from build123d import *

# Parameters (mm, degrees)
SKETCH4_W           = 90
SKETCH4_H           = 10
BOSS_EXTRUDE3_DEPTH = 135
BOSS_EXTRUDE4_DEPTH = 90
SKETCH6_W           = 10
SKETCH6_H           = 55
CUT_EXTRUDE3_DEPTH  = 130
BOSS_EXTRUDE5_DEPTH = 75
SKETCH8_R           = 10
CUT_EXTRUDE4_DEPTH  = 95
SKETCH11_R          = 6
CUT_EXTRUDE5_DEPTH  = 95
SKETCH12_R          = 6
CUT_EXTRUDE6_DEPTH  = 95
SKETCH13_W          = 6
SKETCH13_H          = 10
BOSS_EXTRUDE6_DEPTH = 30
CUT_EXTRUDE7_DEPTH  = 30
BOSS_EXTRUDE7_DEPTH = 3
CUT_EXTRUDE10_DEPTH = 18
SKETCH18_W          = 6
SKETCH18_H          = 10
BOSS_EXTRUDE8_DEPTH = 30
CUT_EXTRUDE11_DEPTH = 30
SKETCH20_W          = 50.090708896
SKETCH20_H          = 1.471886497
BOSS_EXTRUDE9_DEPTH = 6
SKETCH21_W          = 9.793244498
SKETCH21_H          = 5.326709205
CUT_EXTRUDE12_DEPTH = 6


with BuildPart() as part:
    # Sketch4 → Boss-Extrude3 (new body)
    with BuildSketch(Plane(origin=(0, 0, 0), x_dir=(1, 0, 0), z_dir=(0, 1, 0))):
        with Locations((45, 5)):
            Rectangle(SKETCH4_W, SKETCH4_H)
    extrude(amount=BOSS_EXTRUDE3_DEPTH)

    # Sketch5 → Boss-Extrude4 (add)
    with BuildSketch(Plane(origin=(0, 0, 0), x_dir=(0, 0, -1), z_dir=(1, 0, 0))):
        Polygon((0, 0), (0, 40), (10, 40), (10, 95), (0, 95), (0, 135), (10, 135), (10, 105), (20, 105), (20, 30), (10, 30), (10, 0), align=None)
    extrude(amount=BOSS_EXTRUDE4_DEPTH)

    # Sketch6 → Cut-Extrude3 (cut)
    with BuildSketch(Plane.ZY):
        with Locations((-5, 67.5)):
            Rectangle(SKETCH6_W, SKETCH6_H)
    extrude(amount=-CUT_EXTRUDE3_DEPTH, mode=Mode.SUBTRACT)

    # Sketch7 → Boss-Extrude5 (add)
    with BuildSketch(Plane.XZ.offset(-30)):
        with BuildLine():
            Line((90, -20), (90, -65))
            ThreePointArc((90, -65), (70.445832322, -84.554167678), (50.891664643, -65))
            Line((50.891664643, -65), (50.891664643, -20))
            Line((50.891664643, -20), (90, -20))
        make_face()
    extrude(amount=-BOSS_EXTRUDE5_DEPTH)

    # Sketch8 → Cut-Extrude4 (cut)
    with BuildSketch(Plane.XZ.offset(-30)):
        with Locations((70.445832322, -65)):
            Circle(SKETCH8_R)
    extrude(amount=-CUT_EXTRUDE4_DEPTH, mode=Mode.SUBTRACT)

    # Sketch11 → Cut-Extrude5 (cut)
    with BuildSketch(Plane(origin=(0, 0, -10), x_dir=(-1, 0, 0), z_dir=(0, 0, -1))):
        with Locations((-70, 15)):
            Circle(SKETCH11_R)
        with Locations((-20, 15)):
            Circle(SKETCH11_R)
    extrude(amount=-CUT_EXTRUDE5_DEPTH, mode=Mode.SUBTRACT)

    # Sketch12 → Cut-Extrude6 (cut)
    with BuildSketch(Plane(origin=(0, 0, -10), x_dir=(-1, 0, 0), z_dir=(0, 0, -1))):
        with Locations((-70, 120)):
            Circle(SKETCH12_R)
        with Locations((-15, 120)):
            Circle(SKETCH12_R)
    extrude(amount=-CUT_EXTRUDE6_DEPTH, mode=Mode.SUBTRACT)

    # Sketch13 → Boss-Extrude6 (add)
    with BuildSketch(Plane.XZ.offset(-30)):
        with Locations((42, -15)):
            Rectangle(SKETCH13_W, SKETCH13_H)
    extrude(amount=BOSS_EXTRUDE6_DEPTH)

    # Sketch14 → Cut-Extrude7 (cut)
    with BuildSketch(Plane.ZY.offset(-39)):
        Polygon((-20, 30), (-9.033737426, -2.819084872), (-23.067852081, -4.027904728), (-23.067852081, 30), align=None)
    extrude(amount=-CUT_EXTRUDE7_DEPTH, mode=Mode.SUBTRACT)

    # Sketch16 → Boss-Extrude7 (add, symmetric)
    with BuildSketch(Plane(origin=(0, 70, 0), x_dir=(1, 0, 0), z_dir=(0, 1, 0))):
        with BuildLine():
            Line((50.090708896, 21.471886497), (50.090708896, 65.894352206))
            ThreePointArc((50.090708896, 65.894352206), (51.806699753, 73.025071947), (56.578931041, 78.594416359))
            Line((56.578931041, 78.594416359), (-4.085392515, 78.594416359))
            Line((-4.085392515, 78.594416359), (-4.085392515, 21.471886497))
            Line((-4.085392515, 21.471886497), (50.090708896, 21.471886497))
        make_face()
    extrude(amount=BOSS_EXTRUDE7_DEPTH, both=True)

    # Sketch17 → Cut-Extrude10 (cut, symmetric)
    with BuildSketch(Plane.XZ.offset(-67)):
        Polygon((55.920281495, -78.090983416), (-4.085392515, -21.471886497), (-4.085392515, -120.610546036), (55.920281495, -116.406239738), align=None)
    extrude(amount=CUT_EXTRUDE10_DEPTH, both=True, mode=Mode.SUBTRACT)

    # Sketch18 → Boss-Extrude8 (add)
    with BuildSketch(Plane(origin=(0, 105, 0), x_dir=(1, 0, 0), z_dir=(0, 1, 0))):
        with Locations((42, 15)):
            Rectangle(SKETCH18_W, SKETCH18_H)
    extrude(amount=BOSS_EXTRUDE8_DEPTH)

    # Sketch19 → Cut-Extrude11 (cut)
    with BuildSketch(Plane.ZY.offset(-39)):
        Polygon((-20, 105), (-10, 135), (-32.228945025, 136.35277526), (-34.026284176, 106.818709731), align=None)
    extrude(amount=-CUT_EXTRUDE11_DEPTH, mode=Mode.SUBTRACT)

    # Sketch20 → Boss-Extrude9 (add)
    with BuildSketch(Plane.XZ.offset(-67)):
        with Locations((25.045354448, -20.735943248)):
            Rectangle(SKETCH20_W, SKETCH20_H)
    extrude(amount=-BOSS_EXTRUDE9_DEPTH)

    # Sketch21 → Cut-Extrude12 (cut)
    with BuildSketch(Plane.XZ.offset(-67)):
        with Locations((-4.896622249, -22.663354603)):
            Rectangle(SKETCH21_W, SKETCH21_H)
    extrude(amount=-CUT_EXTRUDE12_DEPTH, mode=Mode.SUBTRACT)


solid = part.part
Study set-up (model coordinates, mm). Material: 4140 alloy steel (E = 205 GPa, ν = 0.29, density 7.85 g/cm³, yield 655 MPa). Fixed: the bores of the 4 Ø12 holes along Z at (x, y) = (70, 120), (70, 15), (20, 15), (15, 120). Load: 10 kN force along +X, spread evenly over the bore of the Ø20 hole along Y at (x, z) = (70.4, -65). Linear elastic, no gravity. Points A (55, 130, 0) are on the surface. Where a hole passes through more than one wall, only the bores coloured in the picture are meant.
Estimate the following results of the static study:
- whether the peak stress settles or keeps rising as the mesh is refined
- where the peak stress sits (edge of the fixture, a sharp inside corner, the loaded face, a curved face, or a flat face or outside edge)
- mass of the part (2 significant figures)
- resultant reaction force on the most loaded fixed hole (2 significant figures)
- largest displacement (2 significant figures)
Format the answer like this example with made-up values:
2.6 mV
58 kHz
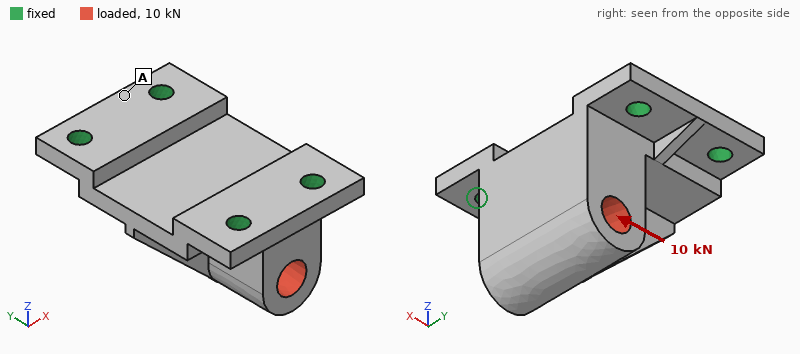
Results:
keeps rising
edge of the fixture
2.3 kg
9.2 kN
84 µm
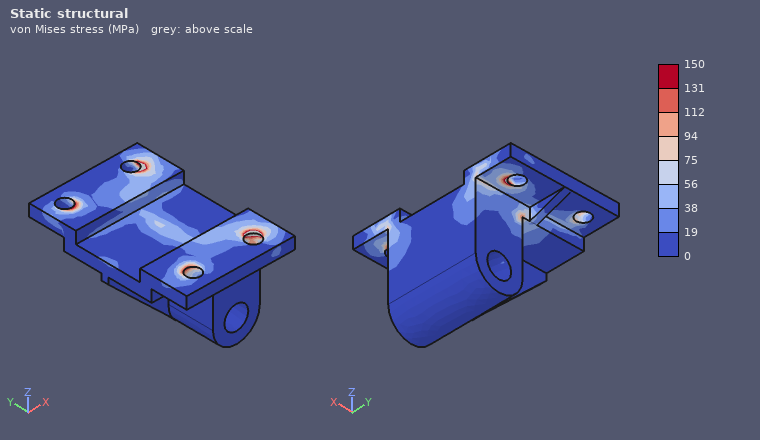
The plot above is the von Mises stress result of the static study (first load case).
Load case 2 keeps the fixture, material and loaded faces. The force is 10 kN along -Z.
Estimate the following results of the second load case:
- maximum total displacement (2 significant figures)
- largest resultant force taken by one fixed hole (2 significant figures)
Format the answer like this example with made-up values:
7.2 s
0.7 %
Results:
15 µm
5.9 kN
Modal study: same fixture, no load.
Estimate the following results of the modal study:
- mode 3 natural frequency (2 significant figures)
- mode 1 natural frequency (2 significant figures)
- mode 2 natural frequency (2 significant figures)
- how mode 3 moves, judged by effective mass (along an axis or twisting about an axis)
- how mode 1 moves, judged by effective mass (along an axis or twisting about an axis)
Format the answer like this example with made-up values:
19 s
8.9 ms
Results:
4200 Hz
2300 Hz
2900 Hz
along Y
along X
